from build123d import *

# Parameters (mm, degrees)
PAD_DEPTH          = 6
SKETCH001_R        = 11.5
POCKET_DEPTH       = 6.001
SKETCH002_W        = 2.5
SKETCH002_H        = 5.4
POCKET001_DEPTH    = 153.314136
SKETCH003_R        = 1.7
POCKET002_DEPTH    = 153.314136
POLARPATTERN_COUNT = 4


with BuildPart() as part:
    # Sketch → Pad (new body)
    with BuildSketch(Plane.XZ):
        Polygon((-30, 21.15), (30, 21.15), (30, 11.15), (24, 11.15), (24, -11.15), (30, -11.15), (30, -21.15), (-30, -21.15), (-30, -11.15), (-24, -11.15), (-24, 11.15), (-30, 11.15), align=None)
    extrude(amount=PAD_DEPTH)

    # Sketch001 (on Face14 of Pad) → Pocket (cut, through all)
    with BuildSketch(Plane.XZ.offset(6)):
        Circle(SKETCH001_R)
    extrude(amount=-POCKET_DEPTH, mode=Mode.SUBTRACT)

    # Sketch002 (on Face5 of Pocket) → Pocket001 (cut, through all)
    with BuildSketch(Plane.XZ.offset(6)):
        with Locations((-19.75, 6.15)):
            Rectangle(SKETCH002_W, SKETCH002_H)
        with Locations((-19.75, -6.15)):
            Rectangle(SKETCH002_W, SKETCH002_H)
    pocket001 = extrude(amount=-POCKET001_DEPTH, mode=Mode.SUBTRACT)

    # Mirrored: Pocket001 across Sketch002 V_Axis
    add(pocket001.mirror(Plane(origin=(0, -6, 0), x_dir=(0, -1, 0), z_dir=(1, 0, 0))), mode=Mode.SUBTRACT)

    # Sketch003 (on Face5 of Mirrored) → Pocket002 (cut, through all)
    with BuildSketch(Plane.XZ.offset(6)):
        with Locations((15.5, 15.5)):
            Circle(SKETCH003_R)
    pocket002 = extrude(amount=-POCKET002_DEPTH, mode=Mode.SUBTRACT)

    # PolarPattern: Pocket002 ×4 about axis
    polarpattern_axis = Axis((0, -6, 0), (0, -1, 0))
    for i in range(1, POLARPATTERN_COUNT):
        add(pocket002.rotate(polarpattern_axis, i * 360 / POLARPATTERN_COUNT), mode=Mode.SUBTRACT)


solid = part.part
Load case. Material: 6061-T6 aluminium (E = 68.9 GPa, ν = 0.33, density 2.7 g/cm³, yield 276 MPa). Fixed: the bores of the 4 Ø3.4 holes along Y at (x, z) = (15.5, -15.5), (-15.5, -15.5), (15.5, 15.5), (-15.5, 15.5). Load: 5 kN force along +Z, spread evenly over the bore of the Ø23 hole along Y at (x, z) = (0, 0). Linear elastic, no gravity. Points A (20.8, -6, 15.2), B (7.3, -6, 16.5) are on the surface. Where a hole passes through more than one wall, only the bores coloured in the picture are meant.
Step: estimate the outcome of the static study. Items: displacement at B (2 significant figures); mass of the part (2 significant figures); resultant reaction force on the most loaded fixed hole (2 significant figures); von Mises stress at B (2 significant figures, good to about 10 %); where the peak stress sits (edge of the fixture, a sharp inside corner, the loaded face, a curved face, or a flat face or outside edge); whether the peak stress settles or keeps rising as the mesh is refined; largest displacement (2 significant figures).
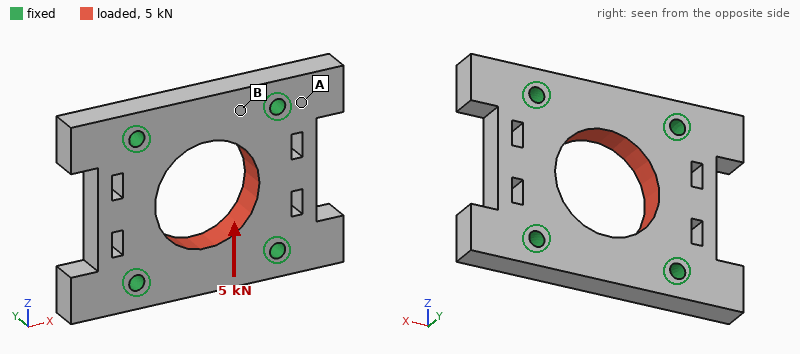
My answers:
4.7 µm
29 g
1.3 kN
15 MPa
edge of the fixture
keeps rising
7.7 µm
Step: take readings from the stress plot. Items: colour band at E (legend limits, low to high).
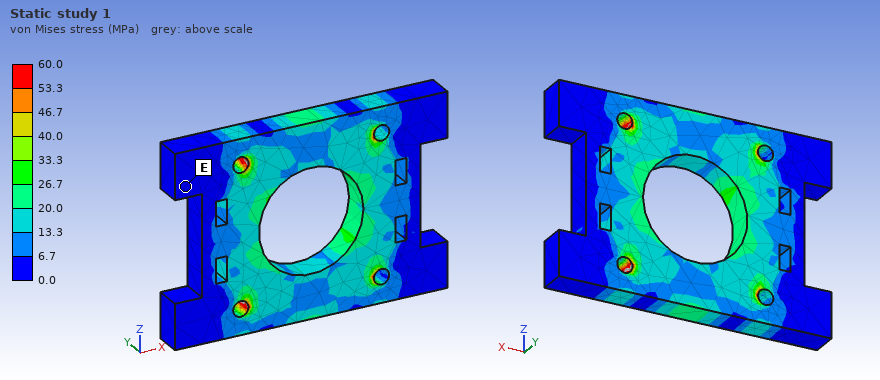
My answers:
0.0 to 6.7 MPa
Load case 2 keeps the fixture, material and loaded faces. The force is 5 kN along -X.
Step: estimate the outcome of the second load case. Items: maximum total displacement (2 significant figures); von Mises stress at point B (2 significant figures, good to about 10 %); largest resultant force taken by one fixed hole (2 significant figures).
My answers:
7.6 µm
13 MPa
1.3 kN
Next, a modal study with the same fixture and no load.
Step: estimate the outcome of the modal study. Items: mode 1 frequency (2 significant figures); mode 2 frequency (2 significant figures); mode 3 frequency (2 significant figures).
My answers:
21 kHz
22 kHz
23 kHz
